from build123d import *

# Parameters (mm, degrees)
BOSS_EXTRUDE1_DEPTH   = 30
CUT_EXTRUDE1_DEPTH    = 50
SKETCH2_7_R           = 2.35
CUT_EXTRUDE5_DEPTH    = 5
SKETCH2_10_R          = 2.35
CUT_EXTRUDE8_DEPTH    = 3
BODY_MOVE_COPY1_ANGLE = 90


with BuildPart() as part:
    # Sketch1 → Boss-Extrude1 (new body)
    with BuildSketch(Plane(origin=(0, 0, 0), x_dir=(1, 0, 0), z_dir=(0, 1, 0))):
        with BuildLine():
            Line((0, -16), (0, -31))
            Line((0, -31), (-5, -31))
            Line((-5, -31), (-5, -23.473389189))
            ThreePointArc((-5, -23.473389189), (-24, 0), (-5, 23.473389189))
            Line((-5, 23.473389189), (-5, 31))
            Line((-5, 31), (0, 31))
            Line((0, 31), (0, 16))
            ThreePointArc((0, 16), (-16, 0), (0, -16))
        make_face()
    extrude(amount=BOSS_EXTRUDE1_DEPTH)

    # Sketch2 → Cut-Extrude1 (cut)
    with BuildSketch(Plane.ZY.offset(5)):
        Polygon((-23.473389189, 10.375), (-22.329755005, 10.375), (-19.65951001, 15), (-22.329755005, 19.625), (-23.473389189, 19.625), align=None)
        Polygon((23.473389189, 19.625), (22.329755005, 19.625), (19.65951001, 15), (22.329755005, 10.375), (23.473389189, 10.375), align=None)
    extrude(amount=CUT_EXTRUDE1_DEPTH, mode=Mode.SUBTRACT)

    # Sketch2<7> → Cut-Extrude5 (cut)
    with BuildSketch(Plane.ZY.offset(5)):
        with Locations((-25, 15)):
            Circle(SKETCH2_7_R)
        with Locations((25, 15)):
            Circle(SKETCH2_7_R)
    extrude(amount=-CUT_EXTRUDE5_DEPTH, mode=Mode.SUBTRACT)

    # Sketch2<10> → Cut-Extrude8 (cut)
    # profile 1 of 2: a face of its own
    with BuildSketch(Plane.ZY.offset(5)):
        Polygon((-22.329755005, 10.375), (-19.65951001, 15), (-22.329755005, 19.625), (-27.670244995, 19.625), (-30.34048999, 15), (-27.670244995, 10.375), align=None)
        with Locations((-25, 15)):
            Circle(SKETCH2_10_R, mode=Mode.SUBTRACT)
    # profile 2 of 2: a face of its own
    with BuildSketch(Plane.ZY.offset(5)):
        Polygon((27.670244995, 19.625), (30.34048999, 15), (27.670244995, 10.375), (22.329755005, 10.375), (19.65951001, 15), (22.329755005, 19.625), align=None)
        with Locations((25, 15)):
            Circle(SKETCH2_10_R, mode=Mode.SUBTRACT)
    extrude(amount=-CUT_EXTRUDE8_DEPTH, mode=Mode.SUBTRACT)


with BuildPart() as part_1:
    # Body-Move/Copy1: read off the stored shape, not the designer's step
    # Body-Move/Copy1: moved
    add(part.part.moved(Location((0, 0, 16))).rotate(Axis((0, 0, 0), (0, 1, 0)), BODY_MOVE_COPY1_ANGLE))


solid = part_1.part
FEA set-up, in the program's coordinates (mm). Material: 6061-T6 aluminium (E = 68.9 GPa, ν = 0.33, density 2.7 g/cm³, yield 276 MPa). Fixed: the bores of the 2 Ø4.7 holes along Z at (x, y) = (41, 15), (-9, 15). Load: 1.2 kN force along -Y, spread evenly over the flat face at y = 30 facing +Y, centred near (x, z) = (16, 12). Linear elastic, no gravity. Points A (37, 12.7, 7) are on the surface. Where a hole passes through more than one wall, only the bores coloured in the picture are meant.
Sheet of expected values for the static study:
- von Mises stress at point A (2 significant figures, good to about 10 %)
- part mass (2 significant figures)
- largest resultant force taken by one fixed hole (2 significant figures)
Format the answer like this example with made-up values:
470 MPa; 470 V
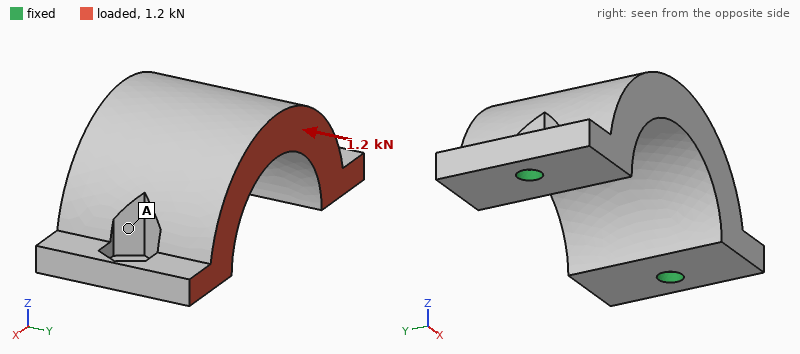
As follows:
31 MPa; 45 g; 600 N
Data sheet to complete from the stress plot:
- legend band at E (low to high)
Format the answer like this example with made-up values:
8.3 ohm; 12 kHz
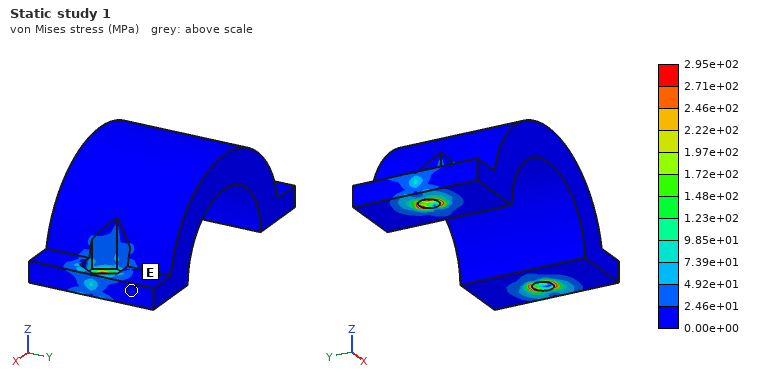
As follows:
0.00e+00 to 2.46e+01 MPa
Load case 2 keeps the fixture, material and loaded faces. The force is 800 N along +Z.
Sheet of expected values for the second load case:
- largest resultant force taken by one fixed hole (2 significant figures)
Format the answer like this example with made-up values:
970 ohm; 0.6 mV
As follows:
450 N
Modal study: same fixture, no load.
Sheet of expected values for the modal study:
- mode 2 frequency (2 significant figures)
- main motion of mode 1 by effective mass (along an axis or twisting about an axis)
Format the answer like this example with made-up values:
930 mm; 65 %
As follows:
10 kHz; along Y
